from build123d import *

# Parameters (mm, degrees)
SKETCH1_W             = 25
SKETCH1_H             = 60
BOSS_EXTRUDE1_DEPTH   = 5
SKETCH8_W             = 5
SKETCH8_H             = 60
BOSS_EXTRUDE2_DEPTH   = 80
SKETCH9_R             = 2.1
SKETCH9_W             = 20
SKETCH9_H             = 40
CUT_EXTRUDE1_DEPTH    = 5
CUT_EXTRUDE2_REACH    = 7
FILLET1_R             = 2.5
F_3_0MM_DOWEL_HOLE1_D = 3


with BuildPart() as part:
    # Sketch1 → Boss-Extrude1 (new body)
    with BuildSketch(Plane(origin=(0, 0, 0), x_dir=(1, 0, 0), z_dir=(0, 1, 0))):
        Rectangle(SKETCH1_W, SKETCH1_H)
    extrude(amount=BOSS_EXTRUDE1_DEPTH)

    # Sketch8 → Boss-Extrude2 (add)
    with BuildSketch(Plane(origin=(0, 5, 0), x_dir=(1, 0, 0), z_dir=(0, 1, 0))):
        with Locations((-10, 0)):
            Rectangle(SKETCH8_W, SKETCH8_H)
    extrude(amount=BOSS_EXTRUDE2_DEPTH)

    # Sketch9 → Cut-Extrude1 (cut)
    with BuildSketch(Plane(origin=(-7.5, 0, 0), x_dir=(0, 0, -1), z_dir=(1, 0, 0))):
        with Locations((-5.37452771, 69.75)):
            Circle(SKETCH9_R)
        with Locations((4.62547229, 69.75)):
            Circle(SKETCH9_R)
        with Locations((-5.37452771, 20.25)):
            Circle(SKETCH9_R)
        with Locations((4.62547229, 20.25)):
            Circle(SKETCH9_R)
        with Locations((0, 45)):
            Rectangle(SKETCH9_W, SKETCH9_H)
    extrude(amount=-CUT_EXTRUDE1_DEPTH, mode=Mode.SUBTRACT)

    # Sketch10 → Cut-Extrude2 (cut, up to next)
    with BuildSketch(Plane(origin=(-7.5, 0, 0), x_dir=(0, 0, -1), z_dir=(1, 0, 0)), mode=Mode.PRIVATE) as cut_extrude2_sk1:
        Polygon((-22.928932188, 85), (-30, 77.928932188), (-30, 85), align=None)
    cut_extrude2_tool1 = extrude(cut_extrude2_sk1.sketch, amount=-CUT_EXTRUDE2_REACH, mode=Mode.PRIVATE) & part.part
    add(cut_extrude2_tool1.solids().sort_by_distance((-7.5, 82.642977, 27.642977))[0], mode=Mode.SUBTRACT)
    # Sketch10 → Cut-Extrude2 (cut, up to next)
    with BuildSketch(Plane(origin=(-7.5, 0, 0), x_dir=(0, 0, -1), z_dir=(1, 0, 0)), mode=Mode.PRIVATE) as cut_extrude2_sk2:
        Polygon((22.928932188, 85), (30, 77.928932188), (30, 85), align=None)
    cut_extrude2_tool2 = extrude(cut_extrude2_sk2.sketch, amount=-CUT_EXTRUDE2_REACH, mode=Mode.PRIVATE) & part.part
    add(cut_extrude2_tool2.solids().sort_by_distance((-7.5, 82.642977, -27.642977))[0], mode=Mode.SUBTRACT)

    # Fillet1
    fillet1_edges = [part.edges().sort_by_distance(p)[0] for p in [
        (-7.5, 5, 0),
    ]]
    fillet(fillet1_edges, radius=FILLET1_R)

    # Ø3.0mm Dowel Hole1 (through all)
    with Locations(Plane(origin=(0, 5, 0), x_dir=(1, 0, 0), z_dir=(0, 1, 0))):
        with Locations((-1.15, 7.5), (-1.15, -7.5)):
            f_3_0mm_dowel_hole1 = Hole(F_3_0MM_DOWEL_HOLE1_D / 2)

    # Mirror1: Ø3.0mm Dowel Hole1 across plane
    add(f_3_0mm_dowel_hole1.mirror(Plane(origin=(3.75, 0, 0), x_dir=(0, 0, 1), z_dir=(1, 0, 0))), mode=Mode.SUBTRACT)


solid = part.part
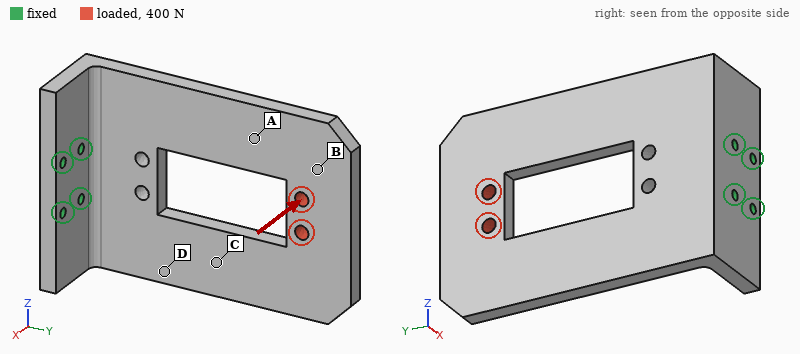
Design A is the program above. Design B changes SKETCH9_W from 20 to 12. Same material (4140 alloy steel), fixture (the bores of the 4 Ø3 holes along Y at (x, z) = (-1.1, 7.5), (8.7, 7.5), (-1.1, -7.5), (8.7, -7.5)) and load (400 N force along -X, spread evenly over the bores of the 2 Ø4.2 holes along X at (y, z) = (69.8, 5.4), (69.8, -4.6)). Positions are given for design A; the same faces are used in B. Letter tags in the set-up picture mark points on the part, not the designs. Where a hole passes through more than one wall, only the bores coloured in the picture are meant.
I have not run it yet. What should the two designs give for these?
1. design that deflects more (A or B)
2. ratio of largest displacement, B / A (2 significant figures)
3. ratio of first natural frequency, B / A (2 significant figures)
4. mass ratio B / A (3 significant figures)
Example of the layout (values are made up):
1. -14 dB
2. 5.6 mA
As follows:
1. A
2. 0.92
3. 1.0
4. 1.06
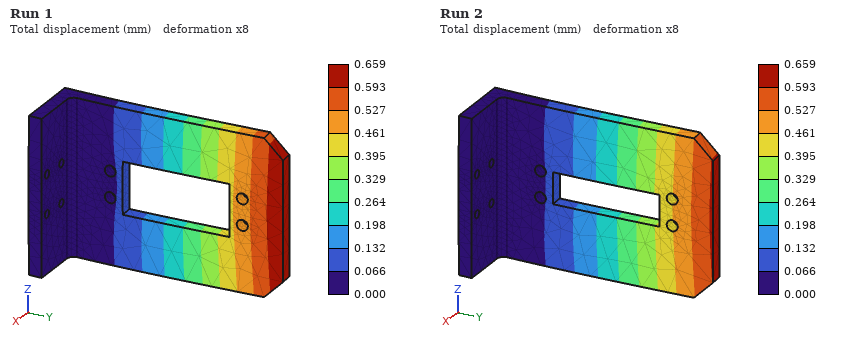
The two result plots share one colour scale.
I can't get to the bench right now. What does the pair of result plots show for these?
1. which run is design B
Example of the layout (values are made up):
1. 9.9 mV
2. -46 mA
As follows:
1. Run 2
